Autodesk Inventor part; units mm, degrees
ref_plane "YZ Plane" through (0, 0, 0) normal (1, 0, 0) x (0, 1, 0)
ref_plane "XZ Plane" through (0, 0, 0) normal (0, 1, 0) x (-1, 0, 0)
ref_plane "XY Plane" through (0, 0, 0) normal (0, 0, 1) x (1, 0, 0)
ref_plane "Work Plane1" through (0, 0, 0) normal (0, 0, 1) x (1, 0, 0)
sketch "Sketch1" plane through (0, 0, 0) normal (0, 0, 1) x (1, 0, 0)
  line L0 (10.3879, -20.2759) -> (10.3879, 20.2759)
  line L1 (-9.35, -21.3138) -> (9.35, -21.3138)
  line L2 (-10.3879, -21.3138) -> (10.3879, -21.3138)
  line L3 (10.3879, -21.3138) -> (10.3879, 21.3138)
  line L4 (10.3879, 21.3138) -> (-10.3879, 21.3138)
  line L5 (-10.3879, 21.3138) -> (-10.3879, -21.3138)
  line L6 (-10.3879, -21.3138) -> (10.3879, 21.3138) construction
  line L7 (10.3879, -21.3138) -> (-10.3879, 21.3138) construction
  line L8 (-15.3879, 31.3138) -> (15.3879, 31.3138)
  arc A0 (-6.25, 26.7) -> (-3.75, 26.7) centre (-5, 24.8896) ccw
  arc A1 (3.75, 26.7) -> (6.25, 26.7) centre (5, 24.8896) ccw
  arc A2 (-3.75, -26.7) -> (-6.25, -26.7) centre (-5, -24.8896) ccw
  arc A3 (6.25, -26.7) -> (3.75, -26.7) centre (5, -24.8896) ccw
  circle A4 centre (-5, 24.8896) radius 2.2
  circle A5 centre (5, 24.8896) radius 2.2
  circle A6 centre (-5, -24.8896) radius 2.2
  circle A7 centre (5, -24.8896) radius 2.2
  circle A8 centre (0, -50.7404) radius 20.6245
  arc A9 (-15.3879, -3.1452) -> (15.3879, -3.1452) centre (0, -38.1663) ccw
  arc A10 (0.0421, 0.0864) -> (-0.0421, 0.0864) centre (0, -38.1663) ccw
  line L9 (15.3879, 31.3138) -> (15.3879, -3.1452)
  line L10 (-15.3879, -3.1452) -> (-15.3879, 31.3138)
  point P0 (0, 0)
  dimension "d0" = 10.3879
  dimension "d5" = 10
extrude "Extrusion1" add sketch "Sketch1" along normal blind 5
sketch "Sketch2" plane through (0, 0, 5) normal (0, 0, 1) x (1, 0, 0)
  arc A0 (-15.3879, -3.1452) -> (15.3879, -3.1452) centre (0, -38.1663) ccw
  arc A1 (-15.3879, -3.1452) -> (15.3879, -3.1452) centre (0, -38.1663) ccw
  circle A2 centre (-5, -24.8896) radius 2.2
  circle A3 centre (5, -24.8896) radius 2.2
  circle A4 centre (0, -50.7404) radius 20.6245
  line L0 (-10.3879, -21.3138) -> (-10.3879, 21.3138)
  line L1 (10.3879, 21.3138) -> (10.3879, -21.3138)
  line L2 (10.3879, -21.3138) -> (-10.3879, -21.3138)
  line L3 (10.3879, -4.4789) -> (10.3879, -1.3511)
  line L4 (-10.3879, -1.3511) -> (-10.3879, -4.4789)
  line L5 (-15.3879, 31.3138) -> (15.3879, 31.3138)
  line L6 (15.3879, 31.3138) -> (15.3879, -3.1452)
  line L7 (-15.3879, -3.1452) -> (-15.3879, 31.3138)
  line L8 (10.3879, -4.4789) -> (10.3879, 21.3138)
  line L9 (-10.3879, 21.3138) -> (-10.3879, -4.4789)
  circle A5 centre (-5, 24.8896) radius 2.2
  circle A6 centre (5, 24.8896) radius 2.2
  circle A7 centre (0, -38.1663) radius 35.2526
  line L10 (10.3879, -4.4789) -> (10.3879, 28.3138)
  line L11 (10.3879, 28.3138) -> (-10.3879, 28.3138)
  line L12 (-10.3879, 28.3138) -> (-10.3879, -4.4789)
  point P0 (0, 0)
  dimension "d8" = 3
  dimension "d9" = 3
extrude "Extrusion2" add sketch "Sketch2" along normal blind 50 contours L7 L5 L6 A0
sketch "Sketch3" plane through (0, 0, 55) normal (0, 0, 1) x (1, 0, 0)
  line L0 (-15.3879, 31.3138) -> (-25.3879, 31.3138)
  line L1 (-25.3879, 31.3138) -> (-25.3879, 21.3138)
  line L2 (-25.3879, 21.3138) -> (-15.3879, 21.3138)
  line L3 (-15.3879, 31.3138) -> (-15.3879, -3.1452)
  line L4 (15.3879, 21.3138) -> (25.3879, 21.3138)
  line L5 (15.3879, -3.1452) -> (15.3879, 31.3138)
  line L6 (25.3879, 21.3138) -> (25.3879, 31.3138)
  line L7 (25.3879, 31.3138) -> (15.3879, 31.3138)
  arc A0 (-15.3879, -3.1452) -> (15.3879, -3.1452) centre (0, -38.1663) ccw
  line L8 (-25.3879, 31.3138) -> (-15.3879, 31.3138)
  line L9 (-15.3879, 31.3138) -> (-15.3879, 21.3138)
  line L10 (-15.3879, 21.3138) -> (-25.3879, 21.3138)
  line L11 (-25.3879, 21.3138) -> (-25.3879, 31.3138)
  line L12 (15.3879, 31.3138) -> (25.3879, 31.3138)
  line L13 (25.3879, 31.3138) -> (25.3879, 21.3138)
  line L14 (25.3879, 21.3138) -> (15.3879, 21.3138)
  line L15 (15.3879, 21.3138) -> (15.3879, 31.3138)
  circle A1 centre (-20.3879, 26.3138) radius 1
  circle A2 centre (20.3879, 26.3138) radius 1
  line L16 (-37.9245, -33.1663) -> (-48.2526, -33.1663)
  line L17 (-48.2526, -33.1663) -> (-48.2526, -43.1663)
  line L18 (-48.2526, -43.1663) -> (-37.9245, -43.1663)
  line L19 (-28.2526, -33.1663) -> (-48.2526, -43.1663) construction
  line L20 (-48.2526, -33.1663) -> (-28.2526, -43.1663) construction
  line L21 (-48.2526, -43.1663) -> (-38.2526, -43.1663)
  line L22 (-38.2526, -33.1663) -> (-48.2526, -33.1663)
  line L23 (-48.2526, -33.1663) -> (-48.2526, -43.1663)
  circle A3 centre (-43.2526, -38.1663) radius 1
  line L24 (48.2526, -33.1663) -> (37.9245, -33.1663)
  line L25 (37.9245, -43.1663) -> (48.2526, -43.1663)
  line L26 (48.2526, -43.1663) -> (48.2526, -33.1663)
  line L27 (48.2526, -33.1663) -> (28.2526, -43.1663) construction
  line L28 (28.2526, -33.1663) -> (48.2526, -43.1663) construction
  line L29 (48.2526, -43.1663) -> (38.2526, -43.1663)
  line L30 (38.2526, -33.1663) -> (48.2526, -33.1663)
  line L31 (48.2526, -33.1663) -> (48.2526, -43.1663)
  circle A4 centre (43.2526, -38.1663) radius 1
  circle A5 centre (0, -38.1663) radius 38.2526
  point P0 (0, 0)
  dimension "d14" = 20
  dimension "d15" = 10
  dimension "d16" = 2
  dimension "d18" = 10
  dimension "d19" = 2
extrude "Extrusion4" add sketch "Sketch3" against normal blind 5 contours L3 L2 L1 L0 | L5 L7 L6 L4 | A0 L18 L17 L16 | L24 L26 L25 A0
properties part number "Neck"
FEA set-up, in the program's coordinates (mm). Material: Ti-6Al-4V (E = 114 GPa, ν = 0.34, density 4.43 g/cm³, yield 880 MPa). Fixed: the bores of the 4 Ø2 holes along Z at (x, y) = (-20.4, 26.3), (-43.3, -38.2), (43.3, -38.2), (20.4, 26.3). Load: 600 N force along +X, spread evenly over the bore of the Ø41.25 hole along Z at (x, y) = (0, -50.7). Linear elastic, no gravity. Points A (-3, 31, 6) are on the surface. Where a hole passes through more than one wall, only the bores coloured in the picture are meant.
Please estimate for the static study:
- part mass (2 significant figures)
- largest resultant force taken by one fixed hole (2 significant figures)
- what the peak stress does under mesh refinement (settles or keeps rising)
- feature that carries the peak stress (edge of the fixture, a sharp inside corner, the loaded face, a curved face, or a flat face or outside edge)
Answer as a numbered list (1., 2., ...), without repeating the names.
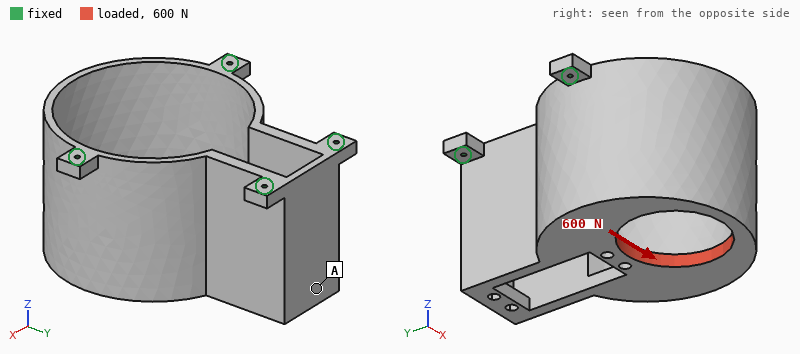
1. 310 g
2. 450 N
3. keeps rising
4. edge of the fixture
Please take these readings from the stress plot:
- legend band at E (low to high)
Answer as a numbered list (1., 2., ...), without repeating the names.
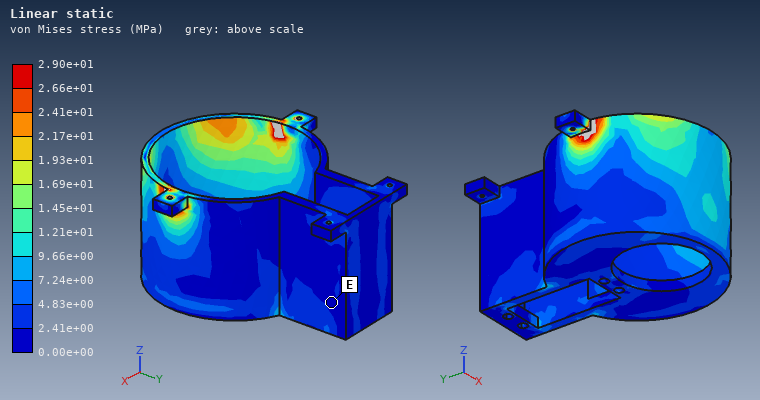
1. 0.00e+00 to 2.41e+00 MPa
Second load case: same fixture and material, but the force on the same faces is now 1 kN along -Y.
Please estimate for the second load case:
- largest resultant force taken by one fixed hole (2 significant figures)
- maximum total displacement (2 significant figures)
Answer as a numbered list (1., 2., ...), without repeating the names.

1. 530 N
2. 28 µm
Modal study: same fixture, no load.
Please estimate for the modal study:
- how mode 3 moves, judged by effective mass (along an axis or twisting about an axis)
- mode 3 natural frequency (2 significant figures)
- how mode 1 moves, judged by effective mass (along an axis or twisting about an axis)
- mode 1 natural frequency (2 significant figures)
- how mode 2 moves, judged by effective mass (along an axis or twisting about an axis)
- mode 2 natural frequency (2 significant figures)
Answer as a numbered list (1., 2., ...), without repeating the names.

1. along X
2. 3000 Hz
3. along X
4. 1800 Hz
5. along Y
6. 2600 Hz
